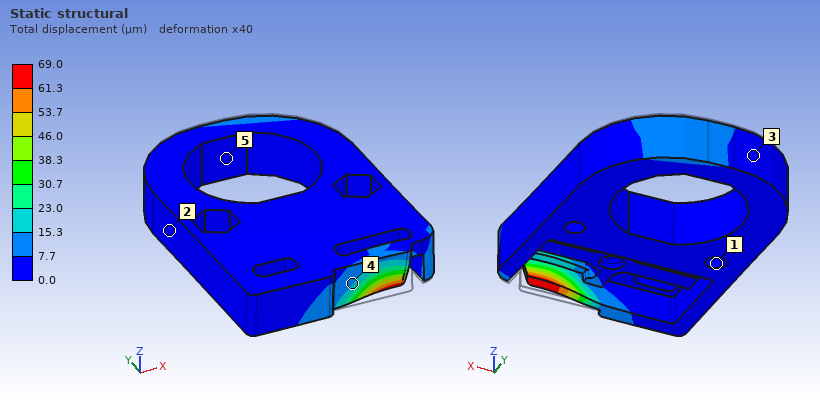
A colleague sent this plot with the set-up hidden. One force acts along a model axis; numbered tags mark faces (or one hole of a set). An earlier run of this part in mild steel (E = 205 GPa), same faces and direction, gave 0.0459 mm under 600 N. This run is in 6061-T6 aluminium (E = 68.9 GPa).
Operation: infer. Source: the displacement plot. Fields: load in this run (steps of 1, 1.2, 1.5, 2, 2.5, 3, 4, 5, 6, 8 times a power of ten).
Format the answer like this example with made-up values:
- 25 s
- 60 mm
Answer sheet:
- 300 N
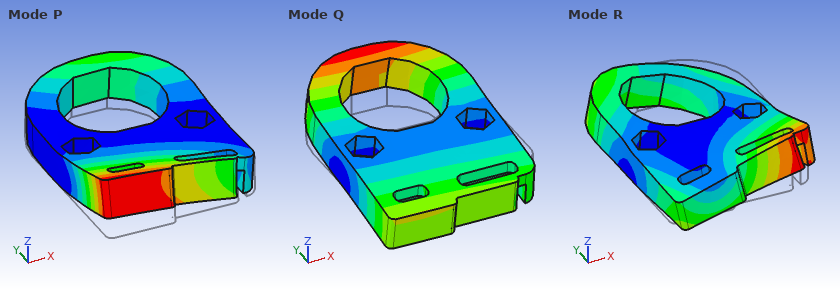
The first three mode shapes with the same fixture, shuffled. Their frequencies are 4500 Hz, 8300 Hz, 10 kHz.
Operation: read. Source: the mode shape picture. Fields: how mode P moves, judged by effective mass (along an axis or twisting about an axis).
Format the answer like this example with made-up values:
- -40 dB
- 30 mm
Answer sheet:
- along Z
